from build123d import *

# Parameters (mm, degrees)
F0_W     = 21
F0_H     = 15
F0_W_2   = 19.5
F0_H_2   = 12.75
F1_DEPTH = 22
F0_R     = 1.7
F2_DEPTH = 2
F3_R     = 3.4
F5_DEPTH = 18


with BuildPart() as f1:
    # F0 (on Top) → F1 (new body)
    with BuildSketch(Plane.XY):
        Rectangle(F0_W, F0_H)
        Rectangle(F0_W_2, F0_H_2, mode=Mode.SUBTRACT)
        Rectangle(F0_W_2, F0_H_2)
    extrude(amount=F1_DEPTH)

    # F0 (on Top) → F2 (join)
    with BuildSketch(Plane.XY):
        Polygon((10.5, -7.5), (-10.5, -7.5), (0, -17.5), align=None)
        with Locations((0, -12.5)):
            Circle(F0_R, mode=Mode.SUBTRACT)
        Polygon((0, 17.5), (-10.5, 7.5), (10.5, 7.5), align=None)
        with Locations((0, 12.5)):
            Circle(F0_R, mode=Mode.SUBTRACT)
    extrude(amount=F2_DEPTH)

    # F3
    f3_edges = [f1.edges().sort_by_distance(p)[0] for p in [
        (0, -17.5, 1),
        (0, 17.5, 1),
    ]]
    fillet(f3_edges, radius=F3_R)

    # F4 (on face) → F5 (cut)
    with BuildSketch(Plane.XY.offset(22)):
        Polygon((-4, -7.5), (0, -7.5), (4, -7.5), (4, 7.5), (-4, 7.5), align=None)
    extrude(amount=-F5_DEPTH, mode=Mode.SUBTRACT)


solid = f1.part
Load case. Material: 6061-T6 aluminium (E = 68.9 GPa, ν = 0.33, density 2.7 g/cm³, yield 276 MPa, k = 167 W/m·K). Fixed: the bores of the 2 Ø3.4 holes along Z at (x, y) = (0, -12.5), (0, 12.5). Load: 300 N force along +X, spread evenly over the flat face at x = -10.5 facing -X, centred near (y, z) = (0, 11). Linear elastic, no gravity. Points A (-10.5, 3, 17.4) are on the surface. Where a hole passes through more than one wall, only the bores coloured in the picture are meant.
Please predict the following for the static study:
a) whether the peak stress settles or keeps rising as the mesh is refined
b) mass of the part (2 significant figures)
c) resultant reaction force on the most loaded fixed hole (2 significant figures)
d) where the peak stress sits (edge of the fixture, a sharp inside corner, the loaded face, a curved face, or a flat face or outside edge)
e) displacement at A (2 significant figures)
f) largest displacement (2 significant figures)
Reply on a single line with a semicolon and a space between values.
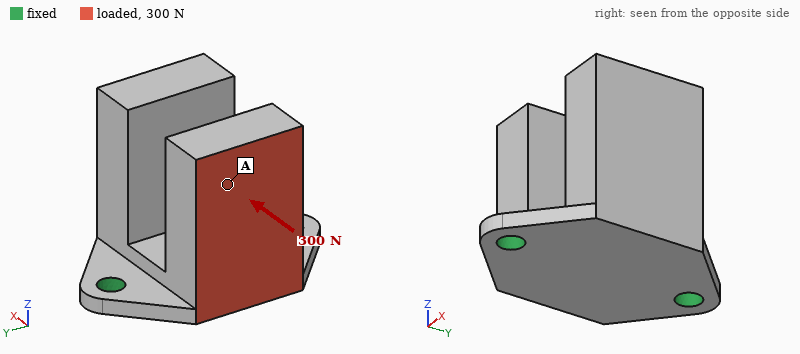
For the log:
keeps rising; 14 g; 160 N; edge of the fixture; 0.14 mm; 0.17 mm
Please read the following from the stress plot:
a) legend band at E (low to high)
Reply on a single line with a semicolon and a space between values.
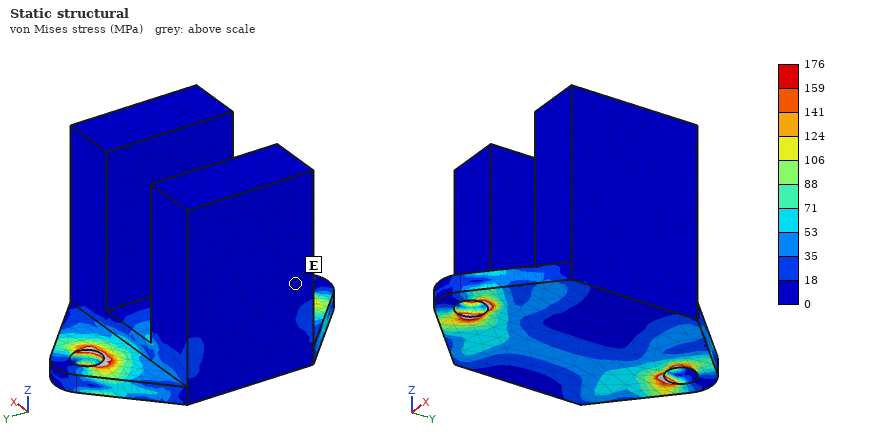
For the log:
0 to 18 MPa
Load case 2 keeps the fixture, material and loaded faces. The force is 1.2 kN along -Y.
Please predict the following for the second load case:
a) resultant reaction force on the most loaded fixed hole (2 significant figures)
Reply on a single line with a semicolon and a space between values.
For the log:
1.0 kN
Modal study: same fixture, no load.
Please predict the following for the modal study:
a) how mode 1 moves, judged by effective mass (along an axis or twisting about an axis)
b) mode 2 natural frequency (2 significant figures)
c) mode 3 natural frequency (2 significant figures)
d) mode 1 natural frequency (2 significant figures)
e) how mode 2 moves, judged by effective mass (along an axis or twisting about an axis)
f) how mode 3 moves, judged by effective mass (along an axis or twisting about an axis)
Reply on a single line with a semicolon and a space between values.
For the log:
along X; 5500 Hz; 7400 Hz; 2400 Hz; along Z; along Y
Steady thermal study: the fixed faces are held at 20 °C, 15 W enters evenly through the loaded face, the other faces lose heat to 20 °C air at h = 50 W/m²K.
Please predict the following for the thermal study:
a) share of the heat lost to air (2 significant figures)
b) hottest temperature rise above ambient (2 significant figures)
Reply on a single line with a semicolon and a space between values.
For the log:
8.8 %; 22 K
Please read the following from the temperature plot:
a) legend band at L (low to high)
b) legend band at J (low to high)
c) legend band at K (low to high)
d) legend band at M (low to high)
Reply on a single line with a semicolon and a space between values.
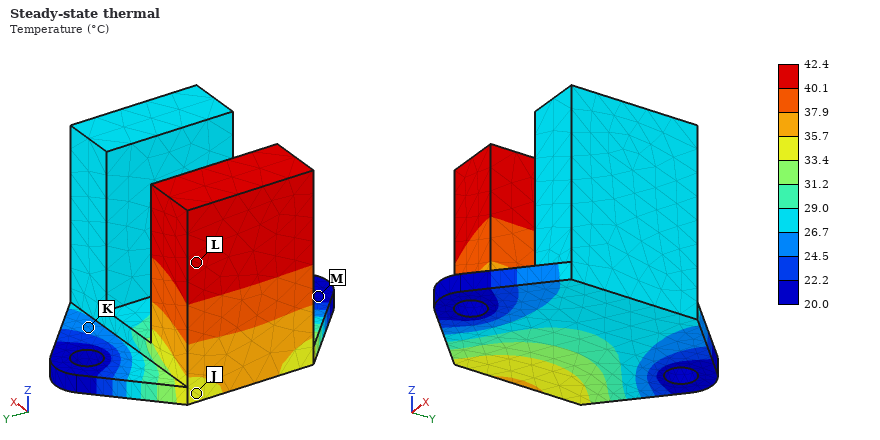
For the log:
40.1 to 42.4 °C; 33.4 to 35.7 °C; 24.5 to 26.7 °C; 20.0 to 22.2 °C
